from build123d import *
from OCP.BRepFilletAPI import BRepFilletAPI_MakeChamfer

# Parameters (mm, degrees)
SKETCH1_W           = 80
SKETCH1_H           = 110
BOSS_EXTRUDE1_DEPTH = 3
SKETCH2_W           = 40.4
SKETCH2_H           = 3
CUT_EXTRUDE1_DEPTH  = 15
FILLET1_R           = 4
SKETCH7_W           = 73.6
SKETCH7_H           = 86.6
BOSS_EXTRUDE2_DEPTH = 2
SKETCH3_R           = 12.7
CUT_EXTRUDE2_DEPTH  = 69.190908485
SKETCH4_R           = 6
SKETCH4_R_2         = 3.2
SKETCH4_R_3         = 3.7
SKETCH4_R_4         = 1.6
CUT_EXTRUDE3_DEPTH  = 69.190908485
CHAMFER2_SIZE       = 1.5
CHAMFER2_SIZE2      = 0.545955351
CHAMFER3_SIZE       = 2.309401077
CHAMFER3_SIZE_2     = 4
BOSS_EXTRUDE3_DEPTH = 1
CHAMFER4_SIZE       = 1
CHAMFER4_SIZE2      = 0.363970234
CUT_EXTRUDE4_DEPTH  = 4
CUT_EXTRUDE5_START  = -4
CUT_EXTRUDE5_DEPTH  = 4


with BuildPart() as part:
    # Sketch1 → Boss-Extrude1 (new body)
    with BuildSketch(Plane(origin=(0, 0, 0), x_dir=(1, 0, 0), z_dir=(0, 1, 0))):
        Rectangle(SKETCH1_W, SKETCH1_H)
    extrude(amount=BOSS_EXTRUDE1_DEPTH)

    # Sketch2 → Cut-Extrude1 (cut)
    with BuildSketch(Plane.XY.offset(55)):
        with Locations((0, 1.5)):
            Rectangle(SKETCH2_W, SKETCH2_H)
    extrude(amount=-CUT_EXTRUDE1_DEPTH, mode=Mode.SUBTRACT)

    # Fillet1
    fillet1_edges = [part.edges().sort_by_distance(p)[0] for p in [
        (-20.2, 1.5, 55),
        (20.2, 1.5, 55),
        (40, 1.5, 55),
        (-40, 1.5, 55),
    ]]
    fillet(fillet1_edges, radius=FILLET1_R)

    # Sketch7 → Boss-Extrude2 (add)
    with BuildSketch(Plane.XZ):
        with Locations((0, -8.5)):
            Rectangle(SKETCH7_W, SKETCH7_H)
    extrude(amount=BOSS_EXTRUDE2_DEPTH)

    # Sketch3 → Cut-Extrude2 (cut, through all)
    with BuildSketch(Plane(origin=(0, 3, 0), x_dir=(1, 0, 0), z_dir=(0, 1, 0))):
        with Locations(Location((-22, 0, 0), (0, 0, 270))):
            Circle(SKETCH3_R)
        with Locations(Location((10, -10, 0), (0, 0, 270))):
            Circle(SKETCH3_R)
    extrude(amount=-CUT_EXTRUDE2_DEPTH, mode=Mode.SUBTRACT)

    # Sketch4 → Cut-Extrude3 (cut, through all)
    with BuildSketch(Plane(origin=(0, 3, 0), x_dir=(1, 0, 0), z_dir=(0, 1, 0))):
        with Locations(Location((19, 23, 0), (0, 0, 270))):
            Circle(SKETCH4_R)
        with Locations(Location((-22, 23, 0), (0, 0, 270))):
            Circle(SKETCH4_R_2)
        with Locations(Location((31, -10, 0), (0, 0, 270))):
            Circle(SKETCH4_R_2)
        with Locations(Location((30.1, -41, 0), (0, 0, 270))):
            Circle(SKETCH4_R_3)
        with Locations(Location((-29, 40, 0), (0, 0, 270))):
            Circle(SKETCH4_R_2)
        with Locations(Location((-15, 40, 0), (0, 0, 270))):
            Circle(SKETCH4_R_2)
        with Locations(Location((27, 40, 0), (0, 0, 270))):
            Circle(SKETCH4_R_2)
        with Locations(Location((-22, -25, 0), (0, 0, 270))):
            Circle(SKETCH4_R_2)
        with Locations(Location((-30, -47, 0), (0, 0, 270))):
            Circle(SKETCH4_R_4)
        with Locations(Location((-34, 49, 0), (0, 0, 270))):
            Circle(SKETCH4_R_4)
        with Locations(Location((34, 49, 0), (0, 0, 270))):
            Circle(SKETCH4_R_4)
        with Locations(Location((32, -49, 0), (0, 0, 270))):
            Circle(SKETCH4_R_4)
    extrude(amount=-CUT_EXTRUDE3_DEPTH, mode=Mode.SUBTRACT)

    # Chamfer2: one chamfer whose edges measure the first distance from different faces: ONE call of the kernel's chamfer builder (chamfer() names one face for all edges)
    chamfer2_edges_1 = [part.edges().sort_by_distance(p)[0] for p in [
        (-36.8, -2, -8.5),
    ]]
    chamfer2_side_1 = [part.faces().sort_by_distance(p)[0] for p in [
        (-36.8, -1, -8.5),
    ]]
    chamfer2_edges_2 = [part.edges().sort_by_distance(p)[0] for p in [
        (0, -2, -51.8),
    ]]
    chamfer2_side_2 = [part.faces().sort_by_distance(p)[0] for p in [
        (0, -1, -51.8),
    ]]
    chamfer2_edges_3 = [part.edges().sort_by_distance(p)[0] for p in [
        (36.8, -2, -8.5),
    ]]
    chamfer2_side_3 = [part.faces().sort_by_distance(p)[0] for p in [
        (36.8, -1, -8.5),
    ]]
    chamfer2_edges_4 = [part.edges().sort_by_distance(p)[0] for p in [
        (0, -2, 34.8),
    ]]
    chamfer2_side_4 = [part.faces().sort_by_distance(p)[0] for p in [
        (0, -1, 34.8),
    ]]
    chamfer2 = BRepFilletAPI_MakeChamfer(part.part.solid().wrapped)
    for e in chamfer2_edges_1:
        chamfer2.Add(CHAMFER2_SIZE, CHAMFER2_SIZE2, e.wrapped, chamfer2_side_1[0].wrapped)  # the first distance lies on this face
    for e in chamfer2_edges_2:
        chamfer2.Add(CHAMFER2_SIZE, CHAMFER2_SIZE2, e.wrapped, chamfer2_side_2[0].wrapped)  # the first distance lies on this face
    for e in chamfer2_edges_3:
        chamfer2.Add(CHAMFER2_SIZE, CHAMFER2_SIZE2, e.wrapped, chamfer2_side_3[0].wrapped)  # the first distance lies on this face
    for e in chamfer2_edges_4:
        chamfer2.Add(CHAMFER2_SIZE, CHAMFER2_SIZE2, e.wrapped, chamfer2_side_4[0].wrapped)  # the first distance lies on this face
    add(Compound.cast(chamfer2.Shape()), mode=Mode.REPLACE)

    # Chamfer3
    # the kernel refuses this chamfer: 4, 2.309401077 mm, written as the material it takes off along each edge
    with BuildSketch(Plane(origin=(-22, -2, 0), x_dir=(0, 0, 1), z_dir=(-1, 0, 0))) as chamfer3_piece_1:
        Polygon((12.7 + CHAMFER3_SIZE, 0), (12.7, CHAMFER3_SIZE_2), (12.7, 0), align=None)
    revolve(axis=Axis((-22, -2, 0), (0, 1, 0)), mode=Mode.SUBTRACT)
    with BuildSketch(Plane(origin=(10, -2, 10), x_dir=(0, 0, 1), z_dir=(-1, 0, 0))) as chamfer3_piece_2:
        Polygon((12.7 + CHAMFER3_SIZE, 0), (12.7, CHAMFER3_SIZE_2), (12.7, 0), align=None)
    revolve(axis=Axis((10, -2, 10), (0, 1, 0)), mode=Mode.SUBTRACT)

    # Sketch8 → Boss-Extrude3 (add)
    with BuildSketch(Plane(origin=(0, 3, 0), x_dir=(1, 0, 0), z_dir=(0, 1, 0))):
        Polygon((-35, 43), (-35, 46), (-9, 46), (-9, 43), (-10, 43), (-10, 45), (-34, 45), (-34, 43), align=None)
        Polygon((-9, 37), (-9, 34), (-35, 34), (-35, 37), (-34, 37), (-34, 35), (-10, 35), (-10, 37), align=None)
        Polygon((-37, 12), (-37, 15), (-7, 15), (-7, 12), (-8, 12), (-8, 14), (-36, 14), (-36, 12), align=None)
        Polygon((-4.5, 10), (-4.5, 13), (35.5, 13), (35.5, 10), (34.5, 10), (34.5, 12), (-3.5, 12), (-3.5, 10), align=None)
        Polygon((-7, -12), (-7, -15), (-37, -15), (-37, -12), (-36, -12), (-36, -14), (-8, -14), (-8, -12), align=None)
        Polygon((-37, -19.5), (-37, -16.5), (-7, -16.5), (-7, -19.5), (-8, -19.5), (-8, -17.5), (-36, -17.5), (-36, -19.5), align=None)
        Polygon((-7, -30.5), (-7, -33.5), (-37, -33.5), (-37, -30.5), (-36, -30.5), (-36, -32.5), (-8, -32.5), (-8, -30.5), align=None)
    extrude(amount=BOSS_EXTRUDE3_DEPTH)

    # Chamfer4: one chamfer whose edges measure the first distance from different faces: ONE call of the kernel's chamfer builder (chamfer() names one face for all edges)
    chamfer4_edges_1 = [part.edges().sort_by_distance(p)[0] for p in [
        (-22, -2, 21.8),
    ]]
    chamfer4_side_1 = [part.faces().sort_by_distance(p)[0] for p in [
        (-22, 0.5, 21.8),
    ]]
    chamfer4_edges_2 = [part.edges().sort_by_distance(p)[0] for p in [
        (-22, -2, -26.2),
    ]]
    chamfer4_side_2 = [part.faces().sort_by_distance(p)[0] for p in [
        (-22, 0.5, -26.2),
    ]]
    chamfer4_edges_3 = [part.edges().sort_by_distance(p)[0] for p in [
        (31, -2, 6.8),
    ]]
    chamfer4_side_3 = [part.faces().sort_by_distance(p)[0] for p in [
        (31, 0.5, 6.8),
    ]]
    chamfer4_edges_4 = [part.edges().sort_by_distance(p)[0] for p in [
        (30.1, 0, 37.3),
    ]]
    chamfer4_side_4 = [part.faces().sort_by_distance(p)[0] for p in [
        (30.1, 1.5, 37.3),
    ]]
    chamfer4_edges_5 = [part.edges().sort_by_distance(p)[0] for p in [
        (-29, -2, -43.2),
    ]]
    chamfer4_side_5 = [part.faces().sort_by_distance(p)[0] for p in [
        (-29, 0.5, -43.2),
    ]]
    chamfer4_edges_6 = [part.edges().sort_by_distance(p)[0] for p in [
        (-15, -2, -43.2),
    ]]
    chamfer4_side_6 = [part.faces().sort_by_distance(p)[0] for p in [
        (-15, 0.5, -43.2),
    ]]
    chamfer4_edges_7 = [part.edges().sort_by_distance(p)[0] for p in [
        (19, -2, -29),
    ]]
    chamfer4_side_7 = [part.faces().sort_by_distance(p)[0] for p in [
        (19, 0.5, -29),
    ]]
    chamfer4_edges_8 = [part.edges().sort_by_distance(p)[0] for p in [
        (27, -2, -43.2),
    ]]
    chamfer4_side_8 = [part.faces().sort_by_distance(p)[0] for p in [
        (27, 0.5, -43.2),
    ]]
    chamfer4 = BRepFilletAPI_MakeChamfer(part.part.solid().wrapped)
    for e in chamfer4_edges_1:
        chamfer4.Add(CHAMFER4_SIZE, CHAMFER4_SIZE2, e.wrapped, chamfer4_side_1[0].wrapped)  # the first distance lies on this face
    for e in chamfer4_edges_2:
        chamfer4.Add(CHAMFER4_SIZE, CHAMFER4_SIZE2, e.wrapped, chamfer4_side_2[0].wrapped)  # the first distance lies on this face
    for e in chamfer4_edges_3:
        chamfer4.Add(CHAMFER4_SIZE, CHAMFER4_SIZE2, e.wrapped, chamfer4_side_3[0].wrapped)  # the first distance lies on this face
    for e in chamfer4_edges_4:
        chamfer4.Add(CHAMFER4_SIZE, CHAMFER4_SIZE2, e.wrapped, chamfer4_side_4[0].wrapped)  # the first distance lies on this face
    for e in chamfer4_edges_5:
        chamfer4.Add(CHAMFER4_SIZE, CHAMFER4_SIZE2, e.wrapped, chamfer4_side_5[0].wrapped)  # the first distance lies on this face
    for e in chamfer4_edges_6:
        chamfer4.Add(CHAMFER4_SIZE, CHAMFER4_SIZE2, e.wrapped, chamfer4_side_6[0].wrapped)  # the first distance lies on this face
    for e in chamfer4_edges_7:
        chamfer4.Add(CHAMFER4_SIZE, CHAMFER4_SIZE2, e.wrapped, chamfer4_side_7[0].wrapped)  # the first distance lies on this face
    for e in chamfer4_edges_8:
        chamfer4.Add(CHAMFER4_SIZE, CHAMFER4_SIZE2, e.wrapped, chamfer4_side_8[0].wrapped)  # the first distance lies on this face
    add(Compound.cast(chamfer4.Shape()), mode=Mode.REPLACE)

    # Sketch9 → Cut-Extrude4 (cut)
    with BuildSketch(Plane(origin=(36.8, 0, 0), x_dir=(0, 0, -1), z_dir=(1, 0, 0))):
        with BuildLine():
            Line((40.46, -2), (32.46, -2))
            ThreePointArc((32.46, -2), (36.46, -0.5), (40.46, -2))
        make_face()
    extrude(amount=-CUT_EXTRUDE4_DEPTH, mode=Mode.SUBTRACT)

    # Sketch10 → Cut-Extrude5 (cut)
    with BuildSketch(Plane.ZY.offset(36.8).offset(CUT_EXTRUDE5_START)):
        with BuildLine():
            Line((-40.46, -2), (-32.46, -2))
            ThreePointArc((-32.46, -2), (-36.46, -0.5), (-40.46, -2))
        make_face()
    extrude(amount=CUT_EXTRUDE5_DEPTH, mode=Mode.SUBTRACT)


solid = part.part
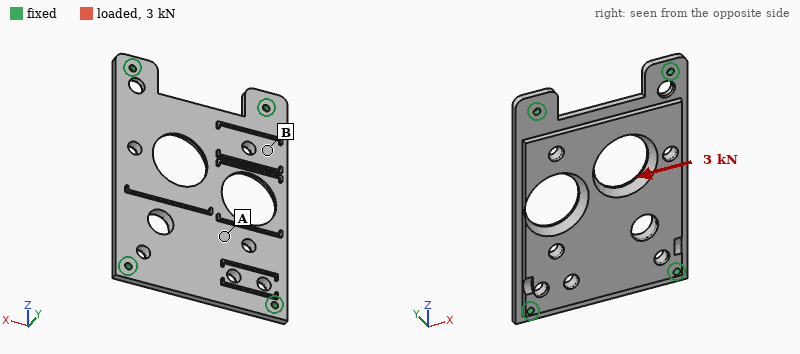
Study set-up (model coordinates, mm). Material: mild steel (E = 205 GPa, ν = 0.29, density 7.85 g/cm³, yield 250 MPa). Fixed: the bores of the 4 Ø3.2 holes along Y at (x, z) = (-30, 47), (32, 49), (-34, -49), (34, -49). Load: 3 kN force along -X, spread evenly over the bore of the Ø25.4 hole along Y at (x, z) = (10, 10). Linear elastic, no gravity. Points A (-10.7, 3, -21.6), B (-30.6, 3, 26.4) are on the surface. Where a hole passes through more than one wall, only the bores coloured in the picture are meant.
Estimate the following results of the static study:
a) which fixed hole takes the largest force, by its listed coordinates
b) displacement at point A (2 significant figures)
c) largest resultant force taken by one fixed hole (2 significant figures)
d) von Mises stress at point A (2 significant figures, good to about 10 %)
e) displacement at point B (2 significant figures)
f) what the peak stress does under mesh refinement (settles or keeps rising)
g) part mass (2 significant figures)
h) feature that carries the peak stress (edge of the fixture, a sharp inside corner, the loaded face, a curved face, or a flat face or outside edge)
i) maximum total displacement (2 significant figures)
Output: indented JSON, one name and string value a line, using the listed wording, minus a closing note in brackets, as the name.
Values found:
{
  "which fixed hole takes the largest force, by its listed coordinates": "(-34, -49)",
  "displacement at point A": "6.2 µm",
  "largest resultant force taken by one fixed hole": "1.2 kN",
  "von Mises stress at point A": "16 MPa",
  "displacement at point B": "8.5 µm",
  "what the peak stress does under mesh refinement": "keeps rising",
  "part mass": "230 g",
  "feature that carries the peak stress": "edge of the fixture",
  "maximum total displacement": "17 µm"
}
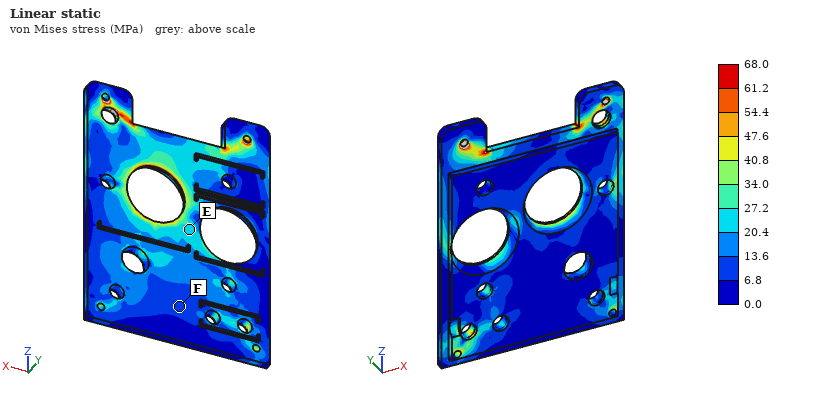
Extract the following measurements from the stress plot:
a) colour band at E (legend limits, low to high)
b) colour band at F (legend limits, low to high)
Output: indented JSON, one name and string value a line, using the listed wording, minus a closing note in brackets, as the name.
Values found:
{
  "colour band at E": "20.4 to 27.2 MPa",
  "colour band at F": "6.8 to 13.6 MPa"
}
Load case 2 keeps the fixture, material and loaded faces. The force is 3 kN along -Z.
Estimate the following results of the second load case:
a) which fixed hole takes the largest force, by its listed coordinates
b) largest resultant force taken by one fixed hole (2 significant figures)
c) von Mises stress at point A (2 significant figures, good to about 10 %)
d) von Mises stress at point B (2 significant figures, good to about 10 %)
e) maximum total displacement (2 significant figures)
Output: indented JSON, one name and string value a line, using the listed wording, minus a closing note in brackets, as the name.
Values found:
{
  "which fixed hole takes the largest force, by its listed coordinates": "(34, -49)",
  "largest resultant force taken by one fixed hole": "1.1 kN",
  "von Mises stress at point A": "9.3 MPa",
  "von Mises stress at point B": "7.5 MPa",
  "maximum total displacement": "10.0 µm"
}
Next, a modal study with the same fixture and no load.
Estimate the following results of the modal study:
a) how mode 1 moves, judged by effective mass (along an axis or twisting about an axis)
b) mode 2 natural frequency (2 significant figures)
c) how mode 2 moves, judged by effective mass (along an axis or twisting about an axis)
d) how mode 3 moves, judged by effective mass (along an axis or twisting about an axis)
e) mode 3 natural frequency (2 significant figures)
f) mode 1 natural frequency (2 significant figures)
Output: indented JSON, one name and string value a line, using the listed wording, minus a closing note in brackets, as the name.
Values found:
{
  "how mode 1 moves, judged by effective mass": "along Y",
  "mode 2 natural frequency": "2800 Hz",
  "how mode 2 moves, judged by effective mass": "twisting about Z",
  "how mode 3 moves, judged by effective mass": "twisting about X",
  "mode 3 natural frequency": "4100 Hz",
  "mode 1 natural frequency": "1600 Hz"
}
